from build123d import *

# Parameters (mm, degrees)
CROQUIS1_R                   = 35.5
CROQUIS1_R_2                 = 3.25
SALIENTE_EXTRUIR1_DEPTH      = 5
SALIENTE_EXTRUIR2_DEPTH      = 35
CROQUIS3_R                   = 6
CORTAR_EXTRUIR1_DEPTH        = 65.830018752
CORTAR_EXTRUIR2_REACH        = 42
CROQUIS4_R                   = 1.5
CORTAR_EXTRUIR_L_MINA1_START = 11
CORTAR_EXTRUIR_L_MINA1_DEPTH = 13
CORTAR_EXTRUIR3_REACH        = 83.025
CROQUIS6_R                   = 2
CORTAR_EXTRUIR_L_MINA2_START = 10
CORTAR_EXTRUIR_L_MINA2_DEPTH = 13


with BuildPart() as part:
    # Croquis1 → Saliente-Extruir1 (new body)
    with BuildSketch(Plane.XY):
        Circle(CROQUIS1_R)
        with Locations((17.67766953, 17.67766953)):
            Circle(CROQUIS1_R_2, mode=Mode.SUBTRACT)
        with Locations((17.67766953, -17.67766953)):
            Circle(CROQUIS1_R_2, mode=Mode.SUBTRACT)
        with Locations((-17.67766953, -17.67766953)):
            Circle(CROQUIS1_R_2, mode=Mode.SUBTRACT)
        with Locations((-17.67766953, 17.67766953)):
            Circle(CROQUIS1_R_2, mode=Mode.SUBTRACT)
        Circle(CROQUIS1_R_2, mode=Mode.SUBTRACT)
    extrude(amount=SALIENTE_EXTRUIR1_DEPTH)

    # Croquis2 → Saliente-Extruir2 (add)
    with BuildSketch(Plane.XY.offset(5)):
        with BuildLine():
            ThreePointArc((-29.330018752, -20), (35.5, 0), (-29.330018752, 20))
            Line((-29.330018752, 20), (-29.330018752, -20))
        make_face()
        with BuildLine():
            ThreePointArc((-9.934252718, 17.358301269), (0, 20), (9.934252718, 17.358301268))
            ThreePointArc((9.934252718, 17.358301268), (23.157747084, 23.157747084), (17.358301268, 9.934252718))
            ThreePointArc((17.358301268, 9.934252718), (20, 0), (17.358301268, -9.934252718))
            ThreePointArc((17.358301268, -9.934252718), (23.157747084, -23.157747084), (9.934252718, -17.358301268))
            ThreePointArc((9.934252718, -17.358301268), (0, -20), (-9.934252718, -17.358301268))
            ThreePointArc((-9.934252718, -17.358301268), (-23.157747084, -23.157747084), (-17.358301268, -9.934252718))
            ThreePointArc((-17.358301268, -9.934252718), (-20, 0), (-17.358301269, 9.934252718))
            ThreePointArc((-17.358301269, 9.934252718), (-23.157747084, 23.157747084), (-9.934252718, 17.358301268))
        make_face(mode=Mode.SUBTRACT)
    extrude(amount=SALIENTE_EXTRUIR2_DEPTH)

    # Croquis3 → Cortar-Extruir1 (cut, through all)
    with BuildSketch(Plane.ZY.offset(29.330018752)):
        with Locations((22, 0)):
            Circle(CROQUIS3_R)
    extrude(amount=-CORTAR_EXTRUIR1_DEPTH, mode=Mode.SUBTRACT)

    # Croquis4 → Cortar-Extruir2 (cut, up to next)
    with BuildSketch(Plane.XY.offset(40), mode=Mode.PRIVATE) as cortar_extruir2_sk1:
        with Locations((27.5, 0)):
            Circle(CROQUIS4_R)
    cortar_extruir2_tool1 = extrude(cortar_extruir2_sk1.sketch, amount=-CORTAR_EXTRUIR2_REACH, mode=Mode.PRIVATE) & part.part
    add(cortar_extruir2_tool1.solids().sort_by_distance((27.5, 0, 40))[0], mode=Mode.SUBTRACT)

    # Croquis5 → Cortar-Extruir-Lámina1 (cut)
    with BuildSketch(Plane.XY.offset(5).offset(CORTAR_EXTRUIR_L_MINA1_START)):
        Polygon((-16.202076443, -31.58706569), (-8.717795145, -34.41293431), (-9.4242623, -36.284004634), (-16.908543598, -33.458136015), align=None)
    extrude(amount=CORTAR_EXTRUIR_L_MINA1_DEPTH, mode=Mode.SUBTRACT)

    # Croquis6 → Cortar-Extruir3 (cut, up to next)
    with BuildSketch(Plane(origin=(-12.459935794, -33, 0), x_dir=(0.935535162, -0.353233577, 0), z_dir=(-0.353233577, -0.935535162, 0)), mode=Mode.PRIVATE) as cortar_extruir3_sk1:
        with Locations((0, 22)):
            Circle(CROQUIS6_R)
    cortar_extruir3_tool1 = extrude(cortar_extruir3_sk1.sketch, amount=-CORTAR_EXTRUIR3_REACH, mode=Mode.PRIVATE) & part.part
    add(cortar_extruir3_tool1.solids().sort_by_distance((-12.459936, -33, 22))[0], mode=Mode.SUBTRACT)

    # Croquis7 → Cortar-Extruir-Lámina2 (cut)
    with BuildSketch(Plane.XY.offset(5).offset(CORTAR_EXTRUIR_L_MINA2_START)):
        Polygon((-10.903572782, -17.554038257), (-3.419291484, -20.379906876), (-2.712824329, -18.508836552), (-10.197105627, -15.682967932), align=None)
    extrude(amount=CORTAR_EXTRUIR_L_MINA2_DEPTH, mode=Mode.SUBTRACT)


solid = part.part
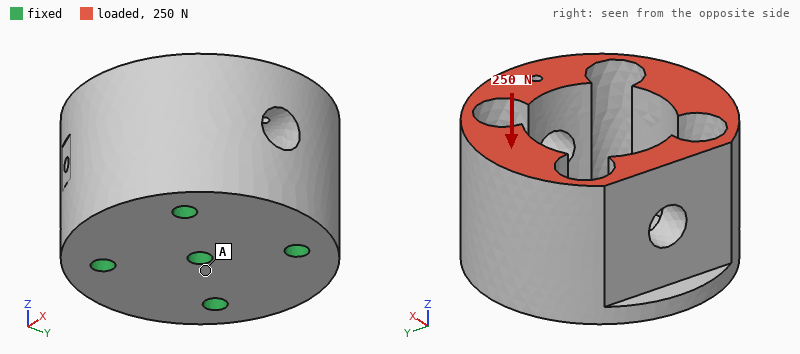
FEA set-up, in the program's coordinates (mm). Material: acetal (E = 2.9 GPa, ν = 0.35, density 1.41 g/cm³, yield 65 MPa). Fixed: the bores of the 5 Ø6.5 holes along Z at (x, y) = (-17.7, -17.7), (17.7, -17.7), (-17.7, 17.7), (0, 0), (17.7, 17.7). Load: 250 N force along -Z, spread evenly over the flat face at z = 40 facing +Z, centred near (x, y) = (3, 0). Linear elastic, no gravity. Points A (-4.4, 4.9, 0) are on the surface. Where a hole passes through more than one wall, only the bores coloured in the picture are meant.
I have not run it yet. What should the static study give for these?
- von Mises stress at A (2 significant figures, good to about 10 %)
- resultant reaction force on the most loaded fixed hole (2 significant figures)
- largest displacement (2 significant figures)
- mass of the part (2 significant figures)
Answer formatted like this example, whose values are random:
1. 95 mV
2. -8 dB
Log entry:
1. 0.21 MPa
2. 69 N
3. 8.6 µm
4. 110 g
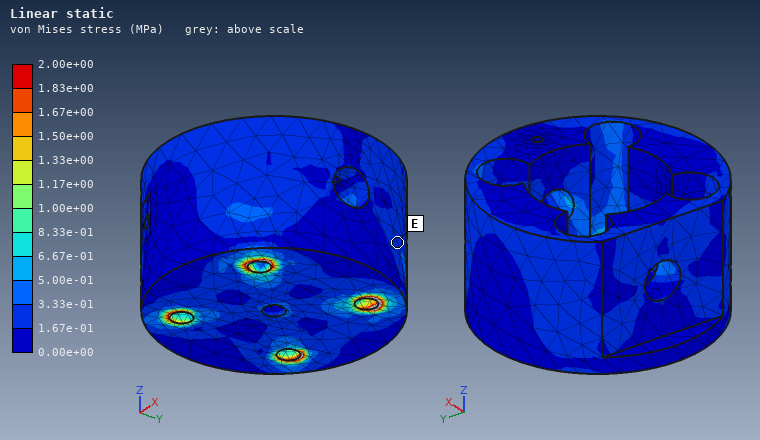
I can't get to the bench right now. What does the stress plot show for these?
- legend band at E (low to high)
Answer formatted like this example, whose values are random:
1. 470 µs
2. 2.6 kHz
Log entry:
1. 1.67e-01 to 3.33e-01 MPa
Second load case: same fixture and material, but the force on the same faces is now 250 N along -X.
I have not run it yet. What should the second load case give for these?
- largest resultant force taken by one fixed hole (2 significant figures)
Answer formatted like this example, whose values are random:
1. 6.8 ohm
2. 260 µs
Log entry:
1. 140 N
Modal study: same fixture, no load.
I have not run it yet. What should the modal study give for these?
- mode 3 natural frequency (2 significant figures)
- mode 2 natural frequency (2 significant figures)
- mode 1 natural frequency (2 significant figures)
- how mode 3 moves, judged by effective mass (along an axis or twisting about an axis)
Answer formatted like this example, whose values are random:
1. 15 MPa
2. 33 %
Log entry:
1. 1700 Hz
2. 1600 Hz
3. 1600 Hz
4. along X
